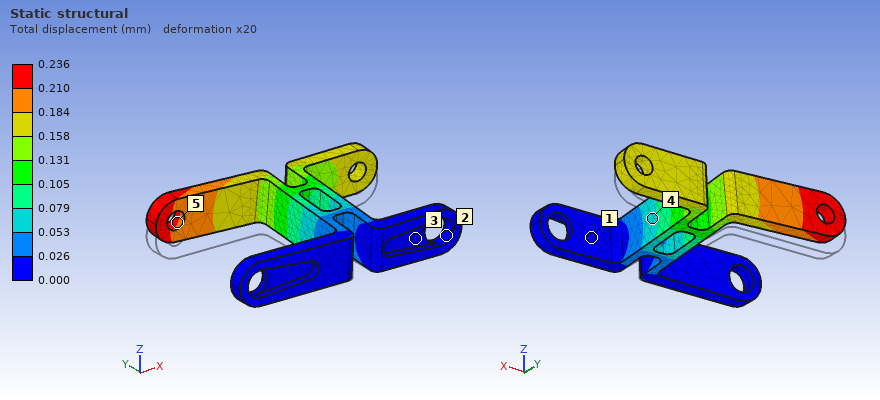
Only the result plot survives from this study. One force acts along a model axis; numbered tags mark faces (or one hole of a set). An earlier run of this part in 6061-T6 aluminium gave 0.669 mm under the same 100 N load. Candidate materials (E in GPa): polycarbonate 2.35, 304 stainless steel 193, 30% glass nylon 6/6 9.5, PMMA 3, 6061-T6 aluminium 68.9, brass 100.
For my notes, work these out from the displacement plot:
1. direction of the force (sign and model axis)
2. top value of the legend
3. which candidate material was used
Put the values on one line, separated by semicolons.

+Z; 0.236 mm; 304 stainless steel
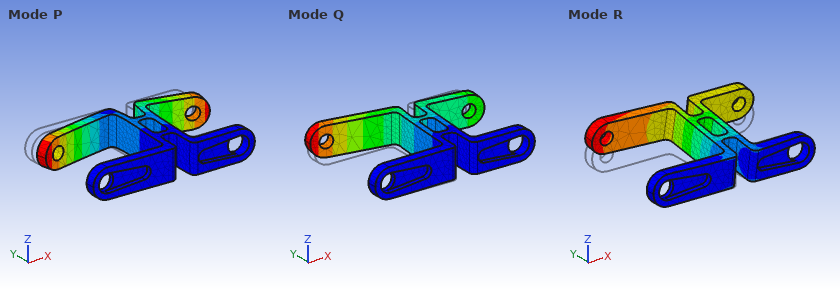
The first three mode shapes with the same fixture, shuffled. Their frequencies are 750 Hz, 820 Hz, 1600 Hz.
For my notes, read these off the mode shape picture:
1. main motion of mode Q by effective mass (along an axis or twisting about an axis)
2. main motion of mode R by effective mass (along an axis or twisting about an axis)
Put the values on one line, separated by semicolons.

along X; along Z
